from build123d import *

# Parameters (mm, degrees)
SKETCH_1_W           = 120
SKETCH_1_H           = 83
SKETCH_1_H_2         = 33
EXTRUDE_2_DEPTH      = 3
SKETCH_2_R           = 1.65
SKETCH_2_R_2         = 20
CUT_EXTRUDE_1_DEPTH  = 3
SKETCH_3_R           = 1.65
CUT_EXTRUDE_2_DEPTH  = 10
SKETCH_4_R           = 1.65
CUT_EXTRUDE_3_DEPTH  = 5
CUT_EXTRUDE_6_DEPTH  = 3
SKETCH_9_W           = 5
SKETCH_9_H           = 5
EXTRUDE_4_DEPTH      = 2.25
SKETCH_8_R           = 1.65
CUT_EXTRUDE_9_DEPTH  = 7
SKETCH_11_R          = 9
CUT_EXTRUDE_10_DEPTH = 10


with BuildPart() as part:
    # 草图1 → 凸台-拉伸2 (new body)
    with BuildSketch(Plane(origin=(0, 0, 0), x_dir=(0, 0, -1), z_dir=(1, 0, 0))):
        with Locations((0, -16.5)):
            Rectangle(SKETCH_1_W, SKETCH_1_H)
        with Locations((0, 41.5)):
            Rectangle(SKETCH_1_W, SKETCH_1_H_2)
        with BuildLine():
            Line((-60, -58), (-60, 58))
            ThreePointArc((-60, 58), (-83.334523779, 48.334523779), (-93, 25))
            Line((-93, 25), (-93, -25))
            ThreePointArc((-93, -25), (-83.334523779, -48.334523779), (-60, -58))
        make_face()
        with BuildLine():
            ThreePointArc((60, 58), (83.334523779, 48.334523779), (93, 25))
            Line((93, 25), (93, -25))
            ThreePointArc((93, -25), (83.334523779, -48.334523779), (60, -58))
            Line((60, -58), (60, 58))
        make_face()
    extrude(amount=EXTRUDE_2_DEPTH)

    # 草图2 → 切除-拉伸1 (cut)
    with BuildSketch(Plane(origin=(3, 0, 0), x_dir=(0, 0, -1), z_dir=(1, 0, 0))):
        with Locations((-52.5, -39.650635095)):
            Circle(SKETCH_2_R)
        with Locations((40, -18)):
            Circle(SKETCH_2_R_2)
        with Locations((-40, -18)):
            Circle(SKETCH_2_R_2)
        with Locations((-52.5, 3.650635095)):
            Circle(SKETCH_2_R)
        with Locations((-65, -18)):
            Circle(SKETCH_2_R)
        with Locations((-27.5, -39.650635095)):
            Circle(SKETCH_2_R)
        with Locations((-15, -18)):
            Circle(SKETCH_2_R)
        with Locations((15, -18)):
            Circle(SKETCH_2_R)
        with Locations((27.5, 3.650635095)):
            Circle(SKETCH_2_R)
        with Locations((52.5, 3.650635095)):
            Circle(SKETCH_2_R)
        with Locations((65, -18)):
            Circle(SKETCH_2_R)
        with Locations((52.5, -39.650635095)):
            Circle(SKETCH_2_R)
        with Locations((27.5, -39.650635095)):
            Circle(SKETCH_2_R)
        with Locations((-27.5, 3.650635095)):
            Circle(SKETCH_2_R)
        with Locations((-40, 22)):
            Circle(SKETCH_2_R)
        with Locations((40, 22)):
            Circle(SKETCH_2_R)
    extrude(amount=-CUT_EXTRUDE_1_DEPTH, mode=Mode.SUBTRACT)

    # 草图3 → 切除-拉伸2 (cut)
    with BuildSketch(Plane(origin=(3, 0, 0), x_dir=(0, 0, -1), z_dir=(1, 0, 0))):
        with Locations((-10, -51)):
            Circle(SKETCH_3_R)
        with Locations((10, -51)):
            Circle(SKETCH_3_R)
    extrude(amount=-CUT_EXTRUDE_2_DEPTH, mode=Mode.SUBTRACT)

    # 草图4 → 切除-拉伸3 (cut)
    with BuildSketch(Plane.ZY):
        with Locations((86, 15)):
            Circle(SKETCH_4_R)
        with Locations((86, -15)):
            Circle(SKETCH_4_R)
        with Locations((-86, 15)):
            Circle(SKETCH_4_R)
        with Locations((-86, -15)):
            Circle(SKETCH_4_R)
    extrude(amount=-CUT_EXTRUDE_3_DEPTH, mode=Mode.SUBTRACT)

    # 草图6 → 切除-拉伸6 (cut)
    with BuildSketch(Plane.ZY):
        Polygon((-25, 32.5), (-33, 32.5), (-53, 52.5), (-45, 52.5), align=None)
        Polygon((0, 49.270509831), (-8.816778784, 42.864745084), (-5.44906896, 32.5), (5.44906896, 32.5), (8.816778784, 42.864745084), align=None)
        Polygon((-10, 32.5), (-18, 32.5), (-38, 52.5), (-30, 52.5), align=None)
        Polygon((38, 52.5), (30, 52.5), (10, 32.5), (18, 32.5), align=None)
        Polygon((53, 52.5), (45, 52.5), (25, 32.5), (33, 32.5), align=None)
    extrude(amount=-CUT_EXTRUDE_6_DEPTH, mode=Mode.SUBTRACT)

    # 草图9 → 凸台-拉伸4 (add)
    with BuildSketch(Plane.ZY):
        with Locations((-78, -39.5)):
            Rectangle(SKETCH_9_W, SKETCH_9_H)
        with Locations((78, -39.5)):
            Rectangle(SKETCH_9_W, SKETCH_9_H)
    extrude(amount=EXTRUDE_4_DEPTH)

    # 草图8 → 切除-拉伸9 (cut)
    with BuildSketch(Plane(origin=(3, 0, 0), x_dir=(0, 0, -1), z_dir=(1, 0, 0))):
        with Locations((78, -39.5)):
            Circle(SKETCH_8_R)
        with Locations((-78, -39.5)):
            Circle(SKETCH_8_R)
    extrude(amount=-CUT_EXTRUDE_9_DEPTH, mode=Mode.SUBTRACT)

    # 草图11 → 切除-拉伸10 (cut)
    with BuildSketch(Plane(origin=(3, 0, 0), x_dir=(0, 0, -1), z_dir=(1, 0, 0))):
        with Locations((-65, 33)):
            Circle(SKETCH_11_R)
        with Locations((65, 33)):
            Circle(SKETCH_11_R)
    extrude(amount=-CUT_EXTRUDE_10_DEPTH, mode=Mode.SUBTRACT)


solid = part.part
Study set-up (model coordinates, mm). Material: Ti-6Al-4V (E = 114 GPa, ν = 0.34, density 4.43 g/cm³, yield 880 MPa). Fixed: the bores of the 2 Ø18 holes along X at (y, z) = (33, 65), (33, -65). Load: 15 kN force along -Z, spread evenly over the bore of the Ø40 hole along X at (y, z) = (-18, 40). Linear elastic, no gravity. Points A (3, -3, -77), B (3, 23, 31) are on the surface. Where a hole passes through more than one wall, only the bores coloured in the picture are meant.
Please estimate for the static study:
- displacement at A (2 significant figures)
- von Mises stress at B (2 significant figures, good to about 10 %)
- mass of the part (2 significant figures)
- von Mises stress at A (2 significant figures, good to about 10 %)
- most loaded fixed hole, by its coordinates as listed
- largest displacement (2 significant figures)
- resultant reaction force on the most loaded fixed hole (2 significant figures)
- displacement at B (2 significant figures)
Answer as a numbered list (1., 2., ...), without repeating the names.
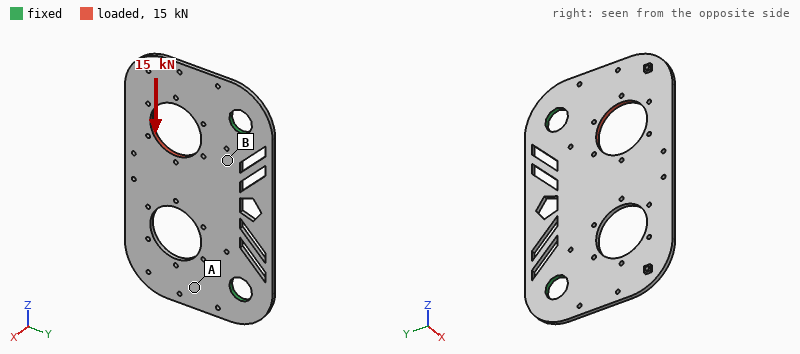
1. 0.031 mm
2. 76 MPa
3. 220 g
4. 30 MPa
5. (33, 65)
6. 0.12 mm
7. 10.0 kN
8. 0.023 mm
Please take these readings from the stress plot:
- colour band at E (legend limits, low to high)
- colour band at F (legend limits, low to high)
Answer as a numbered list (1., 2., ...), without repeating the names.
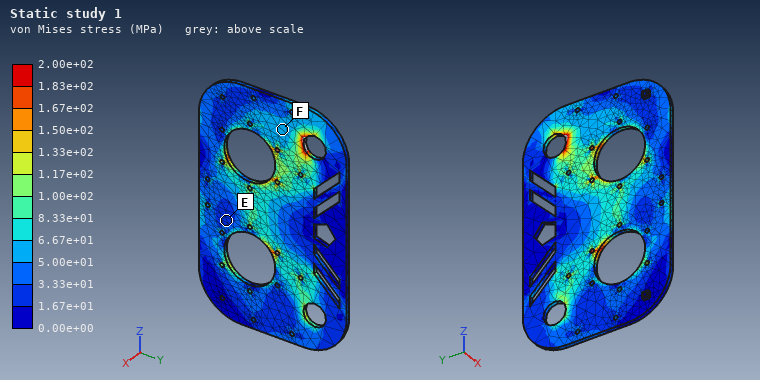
1. 1.67e+01 to 3.33e+01 MPa
2. 5.00e+01 to 6.67e+01 MPa
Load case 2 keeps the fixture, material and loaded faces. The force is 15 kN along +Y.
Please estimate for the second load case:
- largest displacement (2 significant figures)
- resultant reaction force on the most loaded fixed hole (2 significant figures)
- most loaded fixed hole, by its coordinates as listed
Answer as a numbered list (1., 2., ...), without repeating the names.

1. 80 µm
2. 12 kN
3. (33, 65)
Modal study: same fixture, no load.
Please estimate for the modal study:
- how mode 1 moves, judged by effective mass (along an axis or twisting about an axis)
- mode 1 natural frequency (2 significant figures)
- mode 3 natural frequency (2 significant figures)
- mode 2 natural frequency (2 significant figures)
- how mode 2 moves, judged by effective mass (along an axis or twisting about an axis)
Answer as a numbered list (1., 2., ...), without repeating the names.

1. along X
2. 300 Hz
3. 810 Hz
4. 520 Hz
5. twisting about Y
